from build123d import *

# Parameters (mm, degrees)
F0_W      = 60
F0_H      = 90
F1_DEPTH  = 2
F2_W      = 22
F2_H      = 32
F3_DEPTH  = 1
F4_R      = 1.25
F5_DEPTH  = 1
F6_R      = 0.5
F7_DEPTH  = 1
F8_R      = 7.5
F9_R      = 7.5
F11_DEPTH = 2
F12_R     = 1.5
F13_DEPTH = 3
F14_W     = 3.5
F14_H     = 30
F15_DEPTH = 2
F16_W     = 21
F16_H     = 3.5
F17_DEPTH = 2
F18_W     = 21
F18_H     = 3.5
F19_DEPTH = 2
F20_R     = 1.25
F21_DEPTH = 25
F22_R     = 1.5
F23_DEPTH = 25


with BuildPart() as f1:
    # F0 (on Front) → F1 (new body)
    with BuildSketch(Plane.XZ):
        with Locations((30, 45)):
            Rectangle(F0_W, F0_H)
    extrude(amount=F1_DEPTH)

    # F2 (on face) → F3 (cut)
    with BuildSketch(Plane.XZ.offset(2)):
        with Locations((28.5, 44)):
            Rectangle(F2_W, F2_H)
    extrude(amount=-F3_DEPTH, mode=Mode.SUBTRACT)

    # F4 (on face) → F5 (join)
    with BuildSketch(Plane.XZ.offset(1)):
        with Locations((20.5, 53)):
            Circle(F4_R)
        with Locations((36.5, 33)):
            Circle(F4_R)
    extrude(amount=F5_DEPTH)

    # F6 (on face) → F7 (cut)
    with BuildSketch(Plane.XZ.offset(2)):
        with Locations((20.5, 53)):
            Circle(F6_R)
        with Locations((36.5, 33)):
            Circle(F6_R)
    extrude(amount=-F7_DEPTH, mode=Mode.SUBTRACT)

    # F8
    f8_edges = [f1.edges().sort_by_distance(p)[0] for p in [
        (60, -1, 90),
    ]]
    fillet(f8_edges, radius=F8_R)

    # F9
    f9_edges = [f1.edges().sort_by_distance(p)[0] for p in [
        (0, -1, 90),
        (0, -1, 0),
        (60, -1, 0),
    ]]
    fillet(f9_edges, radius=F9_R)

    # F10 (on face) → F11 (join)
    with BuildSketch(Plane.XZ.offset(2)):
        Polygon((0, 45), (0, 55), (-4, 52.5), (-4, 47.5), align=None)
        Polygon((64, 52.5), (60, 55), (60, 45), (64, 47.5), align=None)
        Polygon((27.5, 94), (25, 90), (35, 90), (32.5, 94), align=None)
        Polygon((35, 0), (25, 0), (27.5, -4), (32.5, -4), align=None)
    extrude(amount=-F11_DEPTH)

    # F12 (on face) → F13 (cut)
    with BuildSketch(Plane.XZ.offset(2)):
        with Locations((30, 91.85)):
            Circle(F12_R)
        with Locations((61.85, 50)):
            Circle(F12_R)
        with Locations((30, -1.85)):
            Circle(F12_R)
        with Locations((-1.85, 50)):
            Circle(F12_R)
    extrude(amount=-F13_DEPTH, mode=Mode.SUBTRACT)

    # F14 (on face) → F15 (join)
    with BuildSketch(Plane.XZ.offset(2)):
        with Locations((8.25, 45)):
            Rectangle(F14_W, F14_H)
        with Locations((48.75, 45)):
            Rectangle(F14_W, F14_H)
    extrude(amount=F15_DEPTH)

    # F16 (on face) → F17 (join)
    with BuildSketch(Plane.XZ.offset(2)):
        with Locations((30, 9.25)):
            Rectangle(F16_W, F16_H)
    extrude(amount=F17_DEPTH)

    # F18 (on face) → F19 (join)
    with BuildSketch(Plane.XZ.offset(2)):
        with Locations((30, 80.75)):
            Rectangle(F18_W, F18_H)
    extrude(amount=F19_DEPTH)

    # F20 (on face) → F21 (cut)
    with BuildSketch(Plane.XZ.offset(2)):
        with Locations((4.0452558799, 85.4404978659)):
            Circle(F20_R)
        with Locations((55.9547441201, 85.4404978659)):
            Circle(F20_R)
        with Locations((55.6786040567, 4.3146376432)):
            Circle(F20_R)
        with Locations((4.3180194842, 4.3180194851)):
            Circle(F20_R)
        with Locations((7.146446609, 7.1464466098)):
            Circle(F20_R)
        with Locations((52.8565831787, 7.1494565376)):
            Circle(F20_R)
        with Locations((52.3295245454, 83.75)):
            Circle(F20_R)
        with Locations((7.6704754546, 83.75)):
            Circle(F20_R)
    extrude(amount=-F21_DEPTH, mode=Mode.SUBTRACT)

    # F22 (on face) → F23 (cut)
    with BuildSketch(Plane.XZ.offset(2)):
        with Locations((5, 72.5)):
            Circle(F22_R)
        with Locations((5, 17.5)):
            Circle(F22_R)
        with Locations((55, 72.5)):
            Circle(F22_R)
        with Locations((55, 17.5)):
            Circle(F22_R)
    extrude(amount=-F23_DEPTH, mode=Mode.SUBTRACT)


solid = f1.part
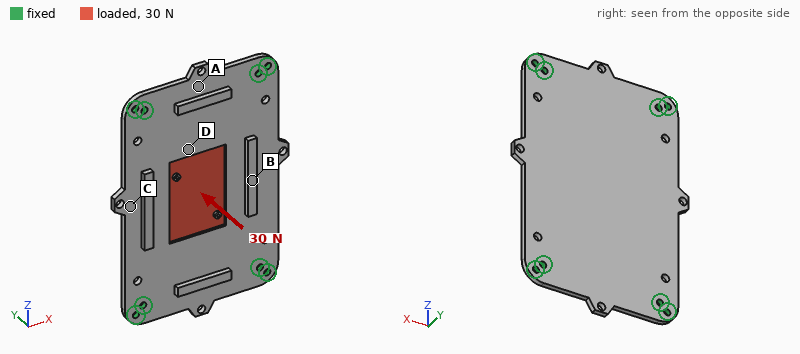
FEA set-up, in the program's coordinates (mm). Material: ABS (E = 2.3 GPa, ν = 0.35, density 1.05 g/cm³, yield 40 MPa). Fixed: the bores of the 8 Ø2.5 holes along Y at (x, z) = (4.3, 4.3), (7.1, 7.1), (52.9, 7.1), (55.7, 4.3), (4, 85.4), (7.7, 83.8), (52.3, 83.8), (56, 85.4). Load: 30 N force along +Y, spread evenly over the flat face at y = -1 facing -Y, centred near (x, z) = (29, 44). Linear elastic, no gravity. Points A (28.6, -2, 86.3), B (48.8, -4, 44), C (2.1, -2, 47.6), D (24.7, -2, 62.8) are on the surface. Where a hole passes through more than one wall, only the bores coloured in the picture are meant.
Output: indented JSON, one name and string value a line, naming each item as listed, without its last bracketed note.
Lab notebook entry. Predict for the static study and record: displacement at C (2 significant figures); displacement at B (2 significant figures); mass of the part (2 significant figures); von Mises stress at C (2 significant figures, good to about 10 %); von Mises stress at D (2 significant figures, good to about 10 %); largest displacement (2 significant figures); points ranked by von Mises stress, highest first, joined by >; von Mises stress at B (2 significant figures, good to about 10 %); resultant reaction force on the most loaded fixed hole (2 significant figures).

{
  "displacement at C": "0.41 mm",
  "displacement at B": "0.59 mm",
  "mass of the part": "11 g",
  "von Mises stress at C": "2.2 MPa",
  "von Mises stress at D": "4.6 MPa",
  "largest displacement": "1.1 mm",
  "points ranked by von Mises stress, highest first, joined by >": "B > D > C > A",
  "von Mises stress at B": "6.8 MPa",
  "resultant reaction force on the most loaded fixed hole": "18 N"
}
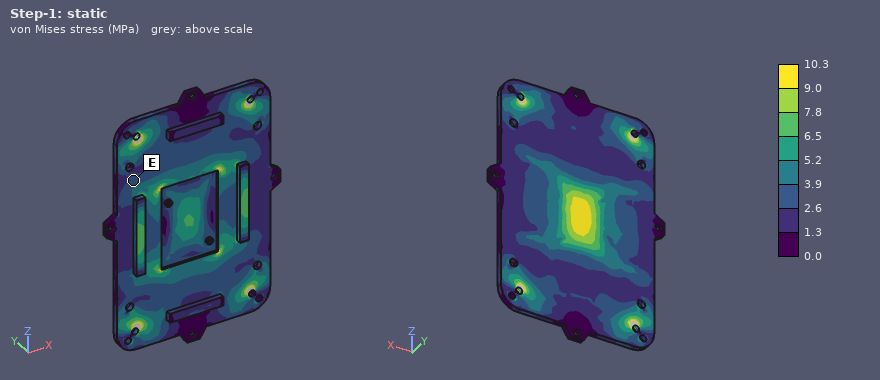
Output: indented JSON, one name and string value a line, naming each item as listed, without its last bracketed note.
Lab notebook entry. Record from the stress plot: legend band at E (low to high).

{
  "legend band at E": "2.6 to 3.9 MPa"
}
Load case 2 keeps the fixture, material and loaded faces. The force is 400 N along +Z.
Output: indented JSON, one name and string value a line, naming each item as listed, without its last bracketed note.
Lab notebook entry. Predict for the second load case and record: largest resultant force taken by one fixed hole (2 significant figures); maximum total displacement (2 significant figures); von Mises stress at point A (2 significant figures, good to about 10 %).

{
  "largest resultant force taken by one fixed hole": "84 N",
  "maximum total displacement": "0.14 mm",
  "von Mises stress at point A": "0.99 MPa"
}
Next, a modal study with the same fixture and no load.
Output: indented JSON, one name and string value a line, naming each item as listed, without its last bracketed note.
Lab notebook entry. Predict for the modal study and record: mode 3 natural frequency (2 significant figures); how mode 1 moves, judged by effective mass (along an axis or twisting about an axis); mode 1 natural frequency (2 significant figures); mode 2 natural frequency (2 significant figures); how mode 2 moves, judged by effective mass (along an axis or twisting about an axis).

{
  "mode 3 natural frequency": "1100 Hz",
  "how mode 1 moves, judged by effective mass": "along Y",
  "mode 1 natural frequency": "510 Hz",
  "mode 2 natural frequency": "680 Hz",
  "how mode 2 moves, judged by effective mass": "twisting about Z"
}
